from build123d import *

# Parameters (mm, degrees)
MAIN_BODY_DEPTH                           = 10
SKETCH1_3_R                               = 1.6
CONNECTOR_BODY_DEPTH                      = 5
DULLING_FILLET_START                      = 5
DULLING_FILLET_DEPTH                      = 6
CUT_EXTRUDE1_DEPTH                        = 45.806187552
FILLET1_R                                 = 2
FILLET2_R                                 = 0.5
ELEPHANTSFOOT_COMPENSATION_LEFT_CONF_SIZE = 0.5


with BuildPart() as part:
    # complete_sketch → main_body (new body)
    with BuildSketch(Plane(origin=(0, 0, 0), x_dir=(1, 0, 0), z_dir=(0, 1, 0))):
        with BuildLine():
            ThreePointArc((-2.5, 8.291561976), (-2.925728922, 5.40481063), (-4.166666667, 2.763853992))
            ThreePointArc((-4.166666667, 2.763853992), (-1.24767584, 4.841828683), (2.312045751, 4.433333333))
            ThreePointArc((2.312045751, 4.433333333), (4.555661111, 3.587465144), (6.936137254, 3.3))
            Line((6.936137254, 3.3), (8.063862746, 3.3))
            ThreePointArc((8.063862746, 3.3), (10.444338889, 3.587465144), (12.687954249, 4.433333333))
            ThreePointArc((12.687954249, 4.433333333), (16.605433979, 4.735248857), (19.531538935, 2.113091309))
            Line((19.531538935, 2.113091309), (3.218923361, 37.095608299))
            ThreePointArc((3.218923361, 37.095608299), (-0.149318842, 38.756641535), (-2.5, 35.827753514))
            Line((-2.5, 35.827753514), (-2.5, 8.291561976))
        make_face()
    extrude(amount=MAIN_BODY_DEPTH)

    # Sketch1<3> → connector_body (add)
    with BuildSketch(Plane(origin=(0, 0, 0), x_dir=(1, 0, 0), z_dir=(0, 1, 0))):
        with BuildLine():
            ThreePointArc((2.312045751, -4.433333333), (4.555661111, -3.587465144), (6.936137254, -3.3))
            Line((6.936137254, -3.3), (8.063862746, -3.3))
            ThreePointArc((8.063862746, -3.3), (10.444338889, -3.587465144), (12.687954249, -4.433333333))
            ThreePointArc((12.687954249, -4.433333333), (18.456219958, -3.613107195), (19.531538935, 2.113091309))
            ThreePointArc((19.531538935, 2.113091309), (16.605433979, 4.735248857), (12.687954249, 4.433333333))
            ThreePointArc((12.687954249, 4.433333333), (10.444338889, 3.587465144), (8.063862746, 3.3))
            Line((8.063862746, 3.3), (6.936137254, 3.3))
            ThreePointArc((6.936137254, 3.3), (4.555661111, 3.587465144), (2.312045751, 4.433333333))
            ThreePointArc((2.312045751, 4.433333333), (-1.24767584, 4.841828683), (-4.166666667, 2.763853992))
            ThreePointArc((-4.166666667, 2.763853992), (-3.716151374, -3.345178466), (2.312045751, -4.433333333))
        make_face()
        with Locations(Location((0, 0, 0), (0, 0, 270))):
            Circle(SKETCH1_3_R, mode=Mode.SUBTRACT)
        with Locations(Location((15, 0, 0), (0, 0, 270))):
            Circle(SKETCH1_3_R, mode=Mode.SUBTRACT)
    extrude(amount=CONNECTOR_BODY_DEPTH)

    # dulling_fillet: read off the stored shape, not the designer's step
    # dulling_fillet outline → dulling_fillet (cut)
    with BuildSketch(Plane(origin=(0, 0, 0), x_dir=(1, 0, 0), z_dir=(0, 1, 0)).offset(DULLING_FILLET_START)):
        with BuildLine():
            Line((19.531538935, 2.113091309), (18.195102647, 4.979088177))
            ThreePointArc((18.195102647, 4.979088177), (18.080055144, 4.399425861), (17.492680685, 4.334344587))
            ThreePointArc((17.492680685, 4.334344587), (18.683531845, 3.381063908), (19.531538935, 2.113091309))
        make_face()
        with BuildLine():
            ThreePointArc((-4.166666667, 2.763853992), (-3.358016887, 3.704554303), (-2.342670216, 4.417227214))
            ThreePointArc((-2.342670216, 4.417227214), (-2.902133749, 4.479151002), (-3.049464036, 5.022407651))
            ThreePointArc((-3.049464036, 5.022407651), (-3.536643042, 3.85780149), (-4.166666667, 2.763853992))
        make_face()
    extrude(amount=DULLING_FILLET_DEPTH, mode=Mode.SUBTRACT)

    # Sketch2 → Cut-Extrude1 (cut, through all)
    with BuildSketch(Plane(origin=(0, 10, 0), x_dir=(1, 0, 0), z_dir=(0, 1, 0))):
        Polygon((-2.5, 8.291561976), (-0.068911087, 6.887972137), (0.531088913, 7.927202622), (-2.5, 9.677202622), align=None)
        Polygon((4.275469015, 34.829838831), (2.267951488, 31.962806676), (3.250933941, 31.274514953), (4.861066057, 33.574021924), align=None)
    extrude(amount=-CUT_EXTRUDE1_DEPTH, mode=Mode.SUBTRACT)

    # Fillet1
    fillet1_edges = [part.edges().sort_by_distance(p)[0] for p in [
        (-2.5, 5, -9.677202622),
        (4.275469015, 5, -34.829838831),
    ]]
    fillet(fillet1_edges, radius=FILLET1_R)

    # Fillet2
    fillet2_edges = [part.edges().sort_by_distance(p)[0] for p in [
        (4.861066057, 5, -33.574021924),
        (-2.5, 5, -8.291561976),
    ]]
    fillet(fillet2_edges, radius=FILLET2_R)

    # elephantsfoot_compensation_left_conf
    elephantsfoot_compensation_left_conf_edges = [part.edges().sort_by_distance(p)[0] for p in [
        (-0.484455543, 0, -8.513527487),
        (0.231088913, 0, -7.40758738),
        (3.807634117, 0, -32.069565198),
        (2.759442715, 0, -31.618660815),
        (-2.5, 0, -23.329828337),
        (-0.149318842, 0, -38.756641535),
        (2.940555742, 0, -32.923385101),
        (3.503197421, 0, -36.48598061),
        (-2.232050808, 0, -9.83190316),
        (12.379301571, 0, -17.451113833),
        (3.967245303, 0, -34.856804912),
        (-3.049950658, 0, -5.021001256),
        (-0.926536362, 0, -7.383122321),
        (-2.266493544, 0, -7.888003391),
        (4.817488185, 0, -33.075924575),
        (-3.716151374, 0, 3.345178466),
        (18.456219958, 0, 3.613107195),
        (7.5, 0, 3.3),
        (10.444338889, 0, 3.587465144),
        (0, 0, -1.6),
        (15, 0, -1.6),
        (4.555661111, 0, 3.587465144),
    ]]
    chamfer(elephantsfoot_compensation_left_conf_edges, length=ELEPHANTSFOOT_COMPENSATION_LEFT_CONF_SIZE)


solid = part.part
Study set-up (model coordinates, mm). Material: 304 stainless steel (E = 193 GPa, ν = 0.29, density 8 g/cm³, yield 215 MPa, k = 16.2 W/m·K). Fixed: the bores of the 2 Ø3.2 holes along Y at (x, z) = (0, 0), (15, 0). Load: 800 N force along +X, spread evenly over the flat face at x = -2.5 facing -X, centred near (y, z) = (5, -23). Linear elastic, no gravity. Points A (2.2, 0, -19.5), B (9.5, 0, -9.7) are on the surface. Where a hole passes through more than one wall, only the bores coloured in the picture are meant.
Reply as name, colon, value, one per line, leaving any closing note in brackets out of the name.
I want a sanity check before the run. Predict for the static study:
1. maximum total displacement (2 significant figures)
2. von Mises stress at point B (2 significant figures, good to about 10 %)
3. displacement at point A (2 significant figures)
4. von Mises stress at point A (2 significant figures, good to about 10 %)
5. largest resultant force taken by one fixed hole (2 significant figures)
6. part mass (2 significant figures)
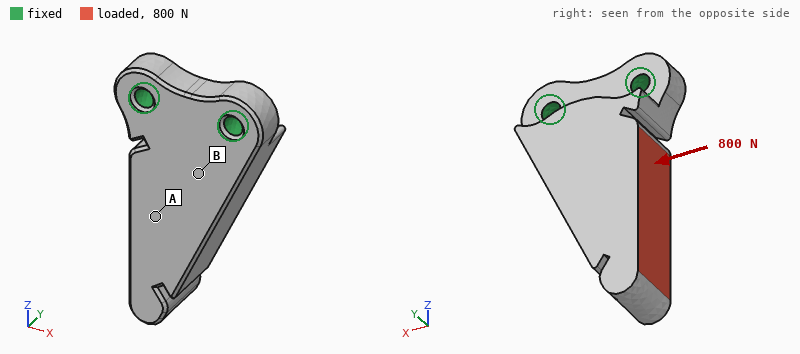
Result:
maximum total displacement: 16 µm
von Mises stress at point B: 19 MPa
displacement at point A: 6.1 µm
von Mises stress at point A: 8.9 MPa
largest resultant force taken by one fixed hole: 1.2 kN
part mass: 42 g
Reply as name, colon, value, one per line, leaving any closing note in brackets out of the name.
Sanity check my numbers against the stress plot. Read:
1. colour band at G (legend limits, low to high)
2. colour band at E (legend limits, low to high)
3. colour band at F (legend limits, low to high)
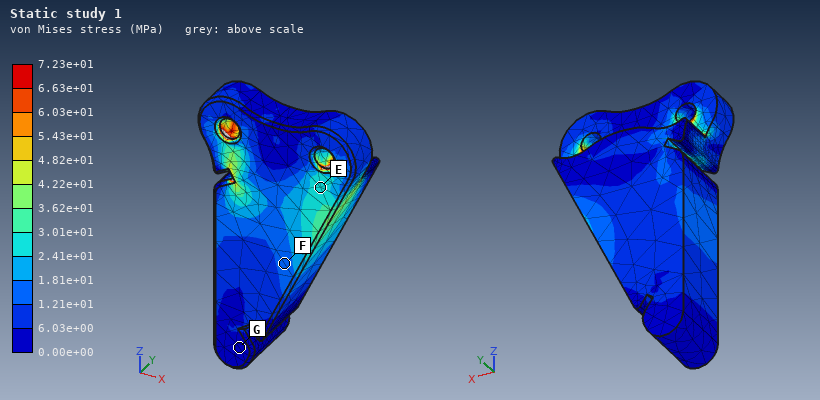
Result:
colour band at G: 0.00e+00 to 6.03e+00 MPa
colour band at E: 2.41e+01 to 3.01e+01 MPa
colour band at F: 1.21e+01 to 1.81e+01 MPa
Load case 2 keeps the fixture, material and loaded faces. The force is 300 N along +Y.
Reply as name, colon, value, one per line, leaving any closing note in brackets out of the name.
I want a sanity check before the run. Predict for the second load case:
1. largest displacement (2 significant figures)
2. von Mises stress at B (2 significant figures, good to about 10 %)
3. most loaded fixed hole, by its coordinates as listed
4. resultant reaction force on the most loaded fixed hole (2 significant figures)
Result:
largest displacement: 44 µm
von Mises stress at B: 24 MPa
most loaded fixed hole, by its coordinates as listed: (0, 0)
resultant reaction force on the most loaded fixed hole: 330 N
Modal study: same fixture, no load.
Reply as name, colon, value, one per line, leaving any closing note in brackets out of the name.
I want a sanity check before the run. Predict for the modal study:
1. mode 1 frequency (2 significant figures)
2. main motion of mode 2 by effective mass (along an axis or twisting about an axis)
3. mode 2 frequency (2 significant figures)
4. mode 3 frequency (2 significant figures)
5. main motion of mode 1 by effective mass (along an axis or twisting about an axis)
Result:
mode 1 frequency: 3500 Hz
main motion of mode 2 by effective mass: along X
mode 2 frequency: 9500 Hz
mode 3 frequency: 21 kHz
main motion of mode 1 by effective mass: along Y
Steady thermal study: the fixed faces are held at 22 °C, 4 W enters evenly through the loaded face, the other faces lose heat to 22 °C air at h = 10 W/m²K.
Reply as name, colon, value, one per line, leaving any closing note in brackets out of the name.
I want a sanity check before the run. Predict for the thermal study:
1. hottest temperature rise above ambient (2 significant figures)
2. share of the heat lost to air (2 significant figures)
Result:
hottest temperature rise above ambient: 48 K
share of the heat lost to air: 12 %
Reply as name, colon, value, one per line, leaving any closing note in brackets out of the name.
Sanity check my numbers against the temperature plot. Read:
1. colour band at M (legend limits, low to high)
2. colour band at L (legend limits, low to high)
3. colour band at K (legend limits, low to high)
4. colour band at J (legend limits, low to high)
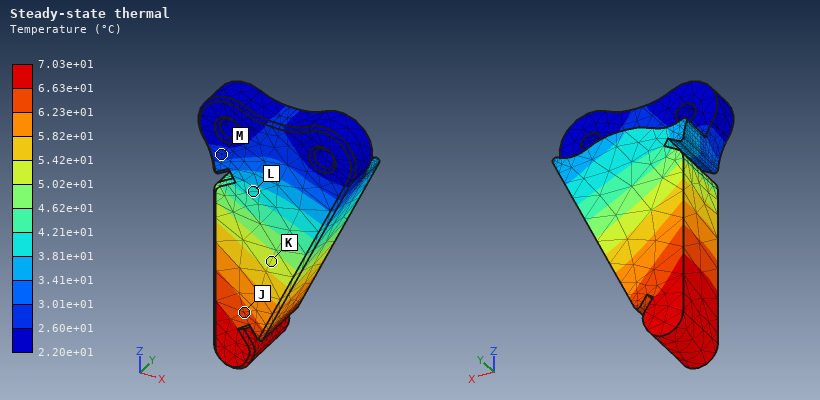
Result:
colour band at M: 2.60e+01 to 3.01e+01 °C
colour band at L: 3.81e+01 to 4.21e+01 °C
colour band at K: 5.02e+01 to 5.42e+01 °C
colour band at J: 6.23e+01 to 6.63e+01 °C
